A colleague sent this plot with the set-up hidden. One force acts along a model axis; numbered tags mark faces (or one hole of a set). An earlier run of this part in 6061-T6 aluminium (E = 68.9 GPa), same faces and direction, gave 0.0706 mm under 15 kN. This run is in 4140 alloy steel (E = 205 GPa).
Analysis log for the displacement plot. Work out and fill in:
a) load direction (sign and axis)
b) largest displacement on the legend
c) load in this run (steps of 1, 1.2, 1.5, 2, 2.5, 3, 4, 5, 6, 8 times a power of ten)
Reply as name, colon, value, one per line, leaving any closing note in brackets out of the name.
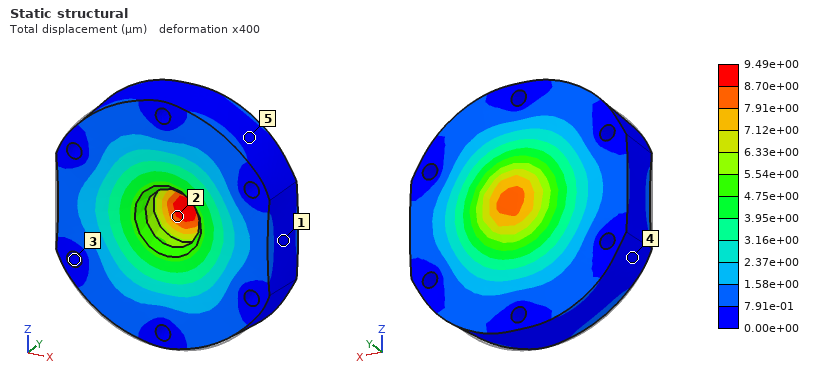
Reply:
load direction: +Y
largest displacement on the legend: 9.49e+00 µm
load in this run: 6 kN
